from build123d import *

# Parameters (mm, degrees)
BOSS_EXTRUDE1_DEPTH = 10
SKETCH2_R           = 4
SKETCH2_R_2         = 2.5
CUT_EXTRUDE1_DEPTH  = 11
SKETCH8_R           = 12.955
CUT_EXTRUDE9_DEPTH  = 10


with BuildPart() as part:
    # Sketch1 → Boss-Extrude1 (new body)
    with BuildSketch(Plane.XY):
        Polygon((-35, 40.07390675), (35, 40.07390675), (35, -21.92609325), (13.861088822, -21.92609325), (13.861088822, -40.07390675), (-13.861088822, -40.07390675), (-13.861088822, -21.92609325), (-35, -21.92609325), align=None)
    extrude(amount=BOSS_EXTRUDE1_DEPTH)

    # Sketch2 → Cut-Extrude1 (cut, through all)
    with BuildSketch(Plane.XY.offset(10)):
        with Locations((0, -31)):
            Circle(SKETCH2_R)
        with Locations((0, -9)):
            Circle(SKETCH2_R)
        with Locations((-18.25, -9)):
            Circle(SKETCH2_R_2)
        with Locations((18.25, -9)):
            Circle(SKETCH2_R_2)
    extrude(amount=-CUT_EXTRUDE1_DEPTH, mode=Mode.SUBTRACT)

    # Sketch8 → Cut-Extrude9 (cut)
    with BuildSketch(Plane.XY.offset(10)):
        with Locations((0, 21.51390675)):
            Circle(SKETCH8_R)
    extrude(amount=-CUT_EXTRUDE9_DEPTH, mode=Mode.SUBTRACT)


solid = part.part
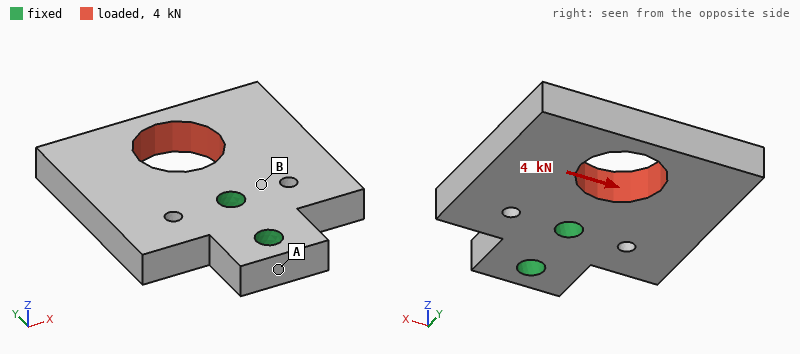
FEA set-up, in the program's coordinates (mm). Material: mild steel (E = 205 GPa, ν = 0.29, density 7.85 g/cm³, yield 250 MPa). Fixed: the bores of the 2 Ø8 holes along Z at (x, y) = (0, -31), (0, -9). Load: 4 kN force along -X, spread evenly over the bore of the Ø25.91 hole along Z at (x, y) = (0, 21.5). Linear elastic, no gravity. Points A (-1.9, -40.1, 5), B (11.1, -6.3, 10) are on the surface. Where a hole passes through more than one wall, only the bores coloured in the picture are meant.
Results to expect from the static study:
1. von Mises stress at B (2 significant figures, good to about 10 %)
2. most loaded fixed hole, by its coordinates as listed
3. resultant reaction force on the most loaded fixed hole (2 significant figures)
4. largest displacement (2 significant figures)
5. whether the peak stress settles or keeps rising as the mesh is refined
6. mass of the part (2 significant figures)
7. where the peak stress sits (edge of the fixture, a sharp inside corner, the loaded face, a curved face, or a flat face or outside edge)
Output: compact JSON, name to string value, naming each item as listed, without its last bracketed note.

{"von Mises stress at B": "22 MPa", "most loaded fixed hole, by its coordinates as listed": "(0, -9)", "resultant reaction force on the most loaded fixed hole": "7.7 kN", "largest displacement": "25 µm", "whether the peak stress settles or keeps rising as the mesh is refined": "keeps rising", "mass of the part": "330 g", "where the peak stress sits": "edge of the fixture"}
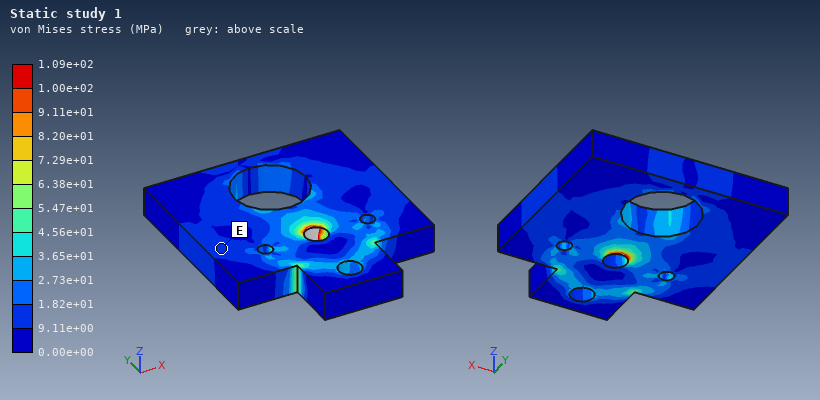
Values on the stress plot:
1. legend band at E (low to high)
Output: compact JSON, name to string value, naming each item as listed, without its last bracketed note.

{"legend band at E": "9.11e+00 to 1.82e+01 MPa"}
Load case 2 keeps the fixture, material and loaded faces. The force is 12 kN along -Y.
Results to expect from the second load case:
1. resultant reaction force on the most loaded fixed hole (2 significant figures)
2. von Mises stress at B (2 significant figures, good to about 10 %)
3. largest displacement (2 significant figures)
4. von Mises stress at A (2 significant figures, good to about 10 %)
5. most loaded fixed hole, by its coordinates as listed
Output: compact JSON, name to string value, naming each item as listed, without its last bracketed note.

{"resultant reaction force on the most loaded fixed hole": "8.7 kN", "von Mises stress at B": "25 MPa", "largest displacement": "17 µm", "von Mises stress at A": "10 MPa", "most loaded fixed hole, by its coordinates as listed": "(0, -9)"}
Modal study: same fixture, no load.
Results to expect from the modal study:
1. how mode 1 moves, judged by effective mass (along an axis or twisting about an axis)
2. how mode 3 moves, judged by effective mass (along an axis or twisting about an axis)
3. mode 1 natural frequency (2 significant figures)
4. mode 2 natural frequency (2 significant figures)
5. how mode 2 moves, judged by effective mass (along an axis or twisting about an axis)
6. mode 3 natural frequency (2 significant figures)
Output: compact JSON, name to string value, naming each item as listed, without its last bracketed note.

{"how mode 1 moves, judged by effective mass": "along Z", "how mode 3 moves, judged by effective mass": "along X", "mode 1 natural frequency": "2800 Hz", "mode 2 natural frequency": "3300 Hz", "how mode 2 moves, judged by effective mass": "twisting about Y", "mode 3 natural frequency": "5300 Hz"}
